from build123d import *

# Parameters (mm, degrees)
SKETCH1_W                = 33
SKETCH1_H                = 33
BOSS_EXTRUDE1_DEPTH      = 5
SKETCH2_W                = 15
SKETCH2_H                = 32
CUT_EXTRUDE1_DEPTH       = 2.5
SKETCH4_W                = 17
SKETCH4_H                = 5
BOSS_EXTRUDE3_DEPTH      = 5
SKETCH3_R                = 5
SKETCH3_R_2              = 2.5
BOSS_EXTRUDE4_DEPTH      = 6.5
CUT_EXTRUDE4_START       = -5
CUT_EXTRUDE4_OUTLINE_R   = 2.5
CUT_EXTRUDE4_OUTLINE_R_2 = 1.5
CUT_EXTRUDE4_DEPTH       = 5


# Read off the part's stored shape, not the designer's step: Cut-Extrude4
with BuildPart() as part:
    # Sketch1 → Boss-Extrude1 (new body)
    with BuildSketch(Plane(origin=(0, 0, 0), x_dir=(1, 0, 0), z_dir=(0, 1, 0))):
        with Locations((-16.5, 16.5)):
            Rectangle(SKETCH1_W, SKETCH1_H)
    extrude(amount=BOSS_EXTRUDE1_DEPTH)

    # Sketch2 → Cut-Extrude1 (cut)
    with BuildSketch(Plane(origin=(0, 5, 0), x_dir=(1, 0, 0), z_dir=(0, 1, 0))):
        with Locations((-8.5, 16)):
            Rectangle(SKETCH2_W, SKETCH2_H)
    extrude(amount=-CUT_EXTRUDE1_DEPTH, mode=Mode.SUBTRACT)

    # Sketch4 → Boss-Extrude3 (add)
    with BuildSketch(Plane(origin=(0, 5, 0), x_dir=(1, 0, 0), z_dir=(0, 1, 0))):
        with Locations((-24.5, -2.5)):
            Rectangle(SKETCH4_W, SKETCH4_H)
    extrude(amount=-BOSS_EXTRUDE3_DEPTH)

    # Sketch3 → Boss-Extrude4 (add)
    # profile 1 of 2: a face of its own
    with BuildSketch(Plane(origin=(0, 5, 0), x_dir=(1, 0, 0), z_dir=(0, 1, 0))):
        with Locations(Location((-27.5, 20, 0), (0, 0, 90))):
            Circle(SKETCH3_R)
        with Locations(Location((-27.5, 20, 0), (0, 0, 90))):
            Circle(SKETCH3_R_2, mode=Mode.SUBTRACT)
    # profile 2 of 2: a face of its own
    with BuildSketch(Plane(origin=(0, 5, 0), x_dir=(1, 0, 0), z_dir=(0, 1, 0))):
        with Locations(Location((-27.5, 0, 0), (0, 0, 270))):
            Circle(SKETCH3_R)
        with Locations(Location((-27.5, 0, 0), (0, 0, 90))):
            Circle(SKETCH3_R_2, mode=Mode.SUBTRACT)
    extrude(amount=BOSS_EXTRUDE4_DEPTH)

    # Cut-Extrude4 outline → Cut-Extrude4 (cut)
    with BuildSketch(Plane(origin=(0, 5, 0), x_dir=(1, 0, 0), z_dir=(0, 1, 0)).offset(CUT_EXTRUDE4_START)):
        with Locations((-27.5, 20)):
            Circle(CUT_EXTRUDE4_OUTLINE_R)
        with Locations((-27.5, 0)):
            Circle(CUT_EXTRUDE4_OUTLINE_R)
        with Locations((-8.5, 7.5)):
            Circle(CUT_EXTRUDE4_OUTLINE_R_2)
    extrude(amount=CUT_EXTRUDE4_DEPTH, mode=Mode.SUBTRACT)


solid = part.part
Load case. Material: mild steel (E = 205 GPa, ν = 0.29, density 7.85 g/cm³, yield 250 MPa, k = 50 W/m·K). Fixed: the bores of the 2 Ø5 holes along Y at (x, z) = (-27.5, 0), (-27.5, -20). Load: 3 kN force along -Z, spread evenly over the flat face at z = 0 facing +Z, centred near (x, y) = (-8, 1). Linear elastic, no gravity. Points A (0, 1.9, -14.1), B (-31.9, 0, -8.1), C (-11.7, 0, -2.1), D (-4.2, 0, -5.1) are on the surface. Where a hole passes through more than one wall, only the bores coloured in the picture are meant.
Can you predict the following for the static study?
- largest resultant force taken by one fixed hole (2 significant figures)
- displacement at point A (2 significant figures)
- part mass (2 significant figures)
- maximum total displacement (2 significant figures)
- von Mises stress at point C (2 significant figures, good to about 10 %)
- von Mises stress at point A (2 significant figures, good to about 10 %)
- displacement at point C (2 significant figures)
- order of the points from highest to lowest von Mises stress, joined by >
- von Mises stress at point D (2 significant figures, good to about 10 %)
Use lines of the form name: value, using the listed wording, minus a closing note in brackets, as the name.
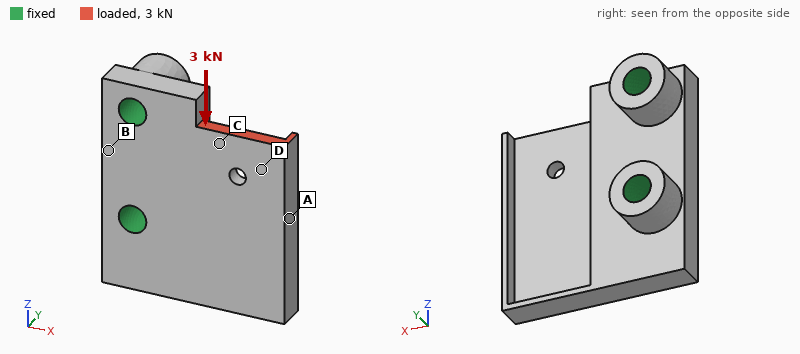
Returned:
largest resultant force taken by one fixed hole: 2.8 kN
displacement at point A: 15 µm
part mass: 41 g
maximum total displacement: 24 µm
von Mises stress at point C: 110 MPa
von Mises stress at point A: 46 MPa
displacement at point C: 11 µm
order of the points from highest to lowest von Mises stress, joined by >: C > D > A > B
von Mises stress at point D: 83 MPa
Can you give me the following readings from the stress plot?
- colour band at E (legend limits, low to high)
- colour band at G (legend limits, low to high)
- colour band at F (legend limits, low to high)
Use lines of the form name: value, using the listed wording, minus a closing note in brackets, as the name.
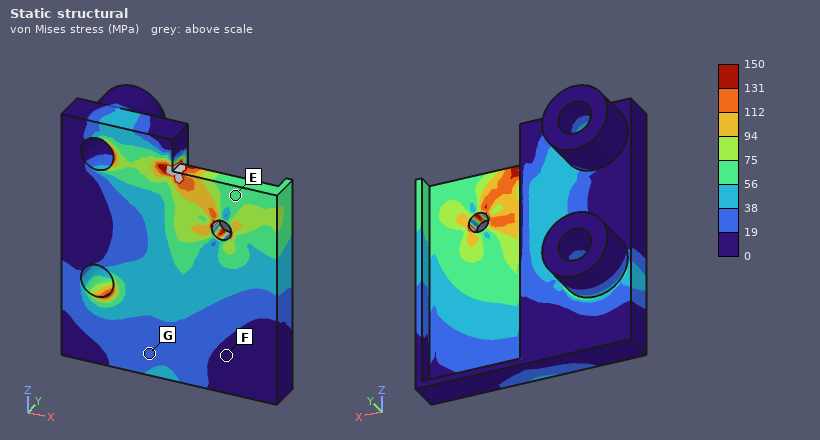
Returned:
colour band at E: 56 to 75 MPa
colour band at G: 19 to 38 MPa
colour band at F: 0 to 19 MPa
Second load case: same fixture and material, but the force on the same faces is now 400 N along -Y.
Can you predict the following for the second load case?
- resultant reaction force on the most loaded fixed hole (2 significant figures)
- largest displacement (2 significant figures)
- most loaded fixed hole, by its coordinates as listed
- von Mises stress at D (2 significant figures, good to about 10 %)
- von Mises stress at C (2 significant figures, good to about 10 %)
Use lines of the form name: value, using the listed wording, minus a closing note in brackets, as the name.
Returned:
resultant reaction force on the most loaded fixed hole: 380 N
largest displacement: 99 µm
most loaded fixed hole, by its coordinates as listed: (-27.5, 0)
von Mises stress at D: 73 MPa
von Mises stress at C: 140 MPa
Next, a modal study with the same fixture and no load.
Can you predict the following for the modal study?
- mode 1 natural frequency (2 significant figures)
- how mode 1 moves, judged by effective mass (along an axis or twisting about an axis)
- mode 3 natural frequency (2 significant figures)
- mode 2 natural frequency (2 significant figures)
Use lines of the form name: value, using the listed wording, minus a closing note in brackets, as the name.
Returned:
mode 1 natural frequency: 5600 Hz
how mode 1 moves, judged by effective mass: along Y
mode 3 natural frequency: 20 kHz
mode 2 natural frequency: 8600 Hz
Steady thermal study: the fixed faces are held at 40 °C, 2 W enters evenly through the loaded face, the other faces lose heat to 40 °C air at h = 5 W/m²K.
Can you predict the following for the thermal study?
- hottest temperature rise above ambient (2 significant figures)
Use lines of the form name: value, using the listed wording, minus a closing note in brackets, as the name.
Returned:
hottest temperature rise above ambient: 15 K
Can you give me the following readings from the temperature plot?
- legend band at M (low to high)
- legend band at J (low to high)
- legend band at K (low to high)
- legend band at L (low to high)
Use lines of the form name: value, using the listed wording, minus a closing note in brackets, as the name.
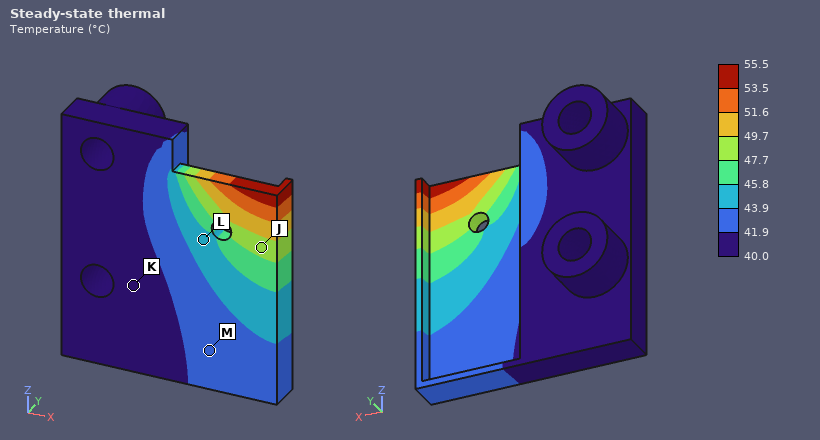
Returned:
legend band at M: 41.9 to 43.9 °C
legend band at J: 47.7 to 49.7 °C
legend band at K: 40.0 to 41.9 °C
legend band at L: 43.9 to 45.8 °C
